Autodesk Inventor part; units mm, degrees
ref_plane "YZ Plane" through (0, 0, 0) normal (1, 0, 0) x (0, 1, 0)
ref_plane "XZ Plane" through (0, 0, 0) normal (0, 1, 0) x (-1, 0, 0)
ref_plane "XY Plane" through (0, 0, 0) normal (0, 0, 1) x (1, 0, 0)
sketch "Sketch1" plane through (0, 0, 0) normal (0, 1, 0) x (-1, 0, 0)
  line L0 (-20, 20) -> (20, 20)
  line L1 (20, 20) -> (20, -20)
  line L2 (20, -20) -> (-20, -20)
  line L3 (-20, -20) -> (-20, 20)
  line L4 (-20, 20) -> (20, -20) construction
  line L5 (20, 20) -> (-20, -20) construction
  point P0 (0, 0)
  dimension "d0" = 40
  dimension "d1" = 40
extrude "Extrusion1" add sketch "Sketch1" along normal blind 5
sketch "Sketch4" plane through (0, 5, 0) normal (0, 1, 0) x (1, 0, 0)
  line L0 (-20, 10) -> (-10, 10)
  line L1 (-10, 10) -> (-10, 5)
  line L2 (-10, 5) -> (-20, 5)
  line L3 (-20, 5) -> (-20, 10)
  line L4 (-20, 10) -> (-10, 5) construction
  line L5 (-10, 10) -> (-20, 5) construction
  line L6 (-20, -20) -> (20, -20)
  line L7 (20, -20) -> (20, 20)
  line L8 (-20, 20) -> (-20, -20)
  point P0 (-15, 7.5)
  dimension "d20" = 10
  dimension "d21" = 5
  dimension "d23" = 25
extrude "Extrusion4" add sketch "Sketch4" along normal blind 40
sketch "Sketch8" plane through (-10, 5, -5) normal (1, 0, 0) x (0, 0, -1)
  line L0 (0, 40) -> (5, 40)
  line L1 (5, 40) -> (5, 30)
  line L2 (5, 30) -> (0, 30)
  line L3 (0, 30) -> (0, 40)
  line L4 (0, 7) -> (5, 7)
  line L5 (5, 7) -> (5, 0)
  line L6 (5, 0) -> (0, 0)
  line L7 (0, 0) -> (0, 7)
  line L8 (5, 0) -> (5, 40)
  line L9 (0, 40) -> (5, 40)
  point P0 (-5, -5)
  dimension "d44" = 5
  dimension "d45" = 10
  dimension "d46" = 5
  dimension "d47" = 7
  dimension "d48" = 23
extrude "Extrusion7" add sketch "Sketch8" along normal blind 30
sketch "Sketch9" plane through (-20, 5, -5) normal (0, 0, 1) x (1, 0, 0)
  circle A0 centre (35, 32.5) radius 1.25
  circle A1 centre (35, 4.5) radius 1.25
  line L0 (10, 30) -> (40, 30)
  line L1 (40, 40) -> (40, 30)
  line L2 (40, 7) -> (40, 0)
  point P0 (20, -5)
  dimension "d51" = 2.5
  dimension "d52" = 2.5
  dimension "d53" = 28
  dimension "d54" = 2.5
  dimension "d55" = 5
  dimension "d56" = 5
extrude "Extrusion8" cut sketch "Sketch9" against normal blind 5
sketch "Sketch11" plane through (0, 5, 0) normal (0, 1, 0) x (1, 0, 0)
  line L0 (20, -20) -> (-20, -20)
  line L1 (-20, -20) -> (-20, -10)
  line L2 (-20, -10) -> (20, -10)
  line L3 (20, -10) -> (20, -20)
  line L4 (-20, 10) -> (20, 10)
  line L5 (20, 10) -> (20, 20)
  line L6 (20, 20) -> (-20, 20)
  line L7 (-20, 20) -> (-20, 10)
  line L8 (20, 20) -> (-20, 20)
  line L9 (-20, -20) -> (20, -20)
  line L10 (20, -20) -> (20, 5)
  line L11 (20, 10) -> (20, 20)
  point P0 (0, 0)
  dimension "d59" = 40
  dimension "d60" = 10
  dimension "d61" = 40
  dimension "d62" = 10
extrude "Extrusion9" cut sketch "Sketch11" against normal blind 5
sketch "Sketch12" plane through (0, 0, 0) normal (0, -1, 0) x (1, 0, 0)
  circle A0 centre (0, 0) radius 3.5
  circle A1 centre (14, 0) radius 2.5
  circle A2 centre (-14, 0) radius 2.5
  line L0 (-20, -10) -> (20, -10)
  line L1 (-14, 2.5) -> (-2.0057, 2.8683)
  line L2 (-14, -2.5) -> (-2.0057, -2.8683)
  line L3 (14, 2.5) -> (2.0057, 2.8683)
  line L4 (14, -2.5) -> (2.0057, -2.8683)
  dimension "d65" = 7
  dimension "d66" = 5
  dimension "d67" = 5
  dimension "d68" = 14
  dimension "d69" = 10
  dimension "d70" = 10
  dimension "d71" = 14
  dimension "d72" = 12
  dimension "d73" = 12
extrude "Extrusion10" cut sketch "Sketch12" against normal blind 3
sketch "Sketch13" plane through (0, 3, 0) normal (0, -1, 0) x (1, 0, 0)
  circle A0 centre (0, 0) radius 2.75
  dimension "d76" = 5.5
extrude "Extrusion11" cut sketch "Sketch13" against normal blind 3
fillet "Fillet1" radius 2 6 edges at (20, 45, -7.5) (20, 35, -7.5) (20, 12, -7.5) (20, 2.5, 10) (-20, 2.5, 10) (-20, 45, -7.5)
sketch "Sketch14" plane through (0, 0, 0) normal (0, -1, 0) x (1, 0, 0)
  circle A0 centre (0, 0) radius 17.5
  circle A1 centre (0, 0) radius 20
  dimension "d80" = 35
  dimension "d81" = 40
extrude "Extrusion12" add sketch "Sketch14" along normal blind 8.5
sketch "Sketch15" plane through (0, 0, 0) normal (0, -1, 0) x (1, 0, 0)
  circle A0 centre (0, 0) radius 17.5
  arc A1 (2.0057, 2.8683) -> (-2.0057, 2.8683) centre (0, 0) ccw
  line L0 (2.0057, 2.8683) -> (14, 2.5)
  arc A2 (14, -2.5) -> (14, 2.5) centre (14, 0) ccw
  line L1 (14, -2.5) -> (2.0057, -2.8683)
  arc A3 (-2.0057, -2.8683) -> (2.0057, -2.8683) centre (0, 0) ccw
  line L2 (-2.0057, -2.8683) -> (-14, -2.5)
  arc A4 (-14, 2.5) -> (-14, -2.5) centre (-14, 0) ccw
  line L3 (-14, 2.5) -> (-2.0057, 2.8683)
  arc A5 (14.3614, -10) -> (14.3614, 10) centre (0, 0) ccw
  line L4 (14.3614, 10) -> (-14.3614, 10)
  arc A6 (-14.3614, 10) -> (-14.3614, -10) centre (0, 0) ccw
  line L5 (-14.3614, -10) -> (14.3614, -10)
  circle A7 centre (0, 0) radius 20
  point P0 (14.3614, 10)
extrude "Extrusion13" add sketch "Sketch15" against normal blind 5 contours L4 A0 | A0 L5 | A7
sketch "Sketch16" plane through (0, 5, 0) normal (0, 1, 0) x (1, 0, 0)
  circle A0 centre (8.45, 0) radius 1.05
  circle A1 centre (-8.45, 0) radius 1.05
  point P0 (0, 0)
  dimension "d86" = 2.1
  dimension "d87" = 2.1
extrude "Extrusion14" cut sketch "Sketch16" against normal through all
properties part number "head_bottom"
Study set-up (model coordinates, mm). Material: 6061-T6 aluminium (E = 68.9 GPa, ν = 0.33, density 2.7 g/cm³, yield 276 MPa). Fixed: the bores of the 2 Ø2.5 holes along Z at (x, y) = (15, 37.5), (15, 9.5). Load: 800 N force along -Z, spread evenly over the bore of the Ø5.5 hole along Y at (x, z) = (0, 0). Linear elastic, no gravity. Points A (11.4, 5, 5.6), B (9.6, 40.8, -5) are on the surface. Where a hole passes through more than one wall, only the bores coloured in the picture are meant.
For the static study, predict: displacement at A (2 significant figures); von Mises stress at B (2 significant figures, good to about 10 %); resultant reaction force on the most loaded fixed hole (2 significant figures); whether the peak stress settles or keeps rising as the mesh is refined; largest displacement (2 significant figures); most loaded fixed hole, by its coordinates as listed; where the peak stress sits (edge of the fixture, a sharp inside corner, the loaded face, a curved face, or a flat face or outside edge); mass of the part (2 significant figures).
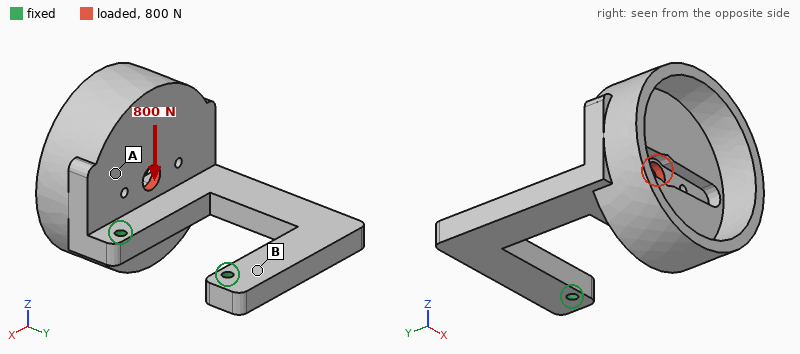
0.088 mm
30 MPa
770 N
keeps rising
0.26 mm
(15, 9.5)
edge of the fixture
35 g
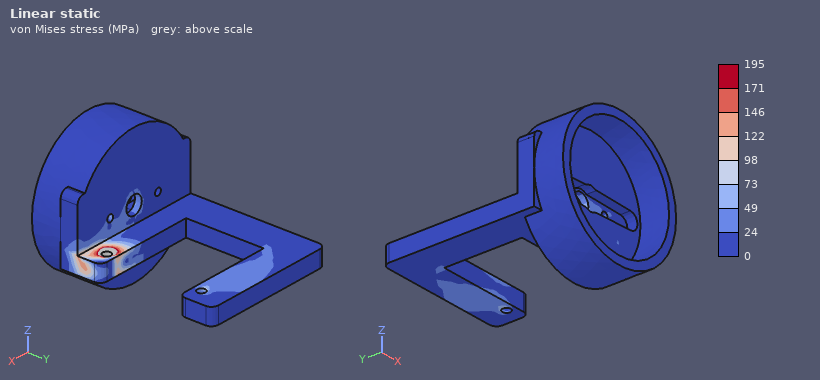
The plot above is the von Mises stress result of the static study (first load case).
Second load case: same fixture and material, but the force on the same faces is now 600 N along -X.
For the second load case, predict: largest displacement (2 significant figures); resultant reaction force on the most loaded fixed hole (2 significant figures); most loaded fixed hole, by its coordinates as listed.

93 µm
650 N
(15, 9.5)
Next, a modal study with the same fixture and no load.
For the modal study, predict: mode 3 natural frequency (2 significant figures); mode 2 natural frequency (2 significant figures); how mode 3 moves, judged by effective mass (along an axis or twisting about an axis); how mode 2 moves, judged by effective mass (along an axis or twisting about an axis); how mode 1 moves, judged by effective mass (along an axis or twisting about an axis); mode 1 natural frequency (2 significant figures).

3700 Hz
2500 Hz
along Y
along Y
along Z
1700 Hz
